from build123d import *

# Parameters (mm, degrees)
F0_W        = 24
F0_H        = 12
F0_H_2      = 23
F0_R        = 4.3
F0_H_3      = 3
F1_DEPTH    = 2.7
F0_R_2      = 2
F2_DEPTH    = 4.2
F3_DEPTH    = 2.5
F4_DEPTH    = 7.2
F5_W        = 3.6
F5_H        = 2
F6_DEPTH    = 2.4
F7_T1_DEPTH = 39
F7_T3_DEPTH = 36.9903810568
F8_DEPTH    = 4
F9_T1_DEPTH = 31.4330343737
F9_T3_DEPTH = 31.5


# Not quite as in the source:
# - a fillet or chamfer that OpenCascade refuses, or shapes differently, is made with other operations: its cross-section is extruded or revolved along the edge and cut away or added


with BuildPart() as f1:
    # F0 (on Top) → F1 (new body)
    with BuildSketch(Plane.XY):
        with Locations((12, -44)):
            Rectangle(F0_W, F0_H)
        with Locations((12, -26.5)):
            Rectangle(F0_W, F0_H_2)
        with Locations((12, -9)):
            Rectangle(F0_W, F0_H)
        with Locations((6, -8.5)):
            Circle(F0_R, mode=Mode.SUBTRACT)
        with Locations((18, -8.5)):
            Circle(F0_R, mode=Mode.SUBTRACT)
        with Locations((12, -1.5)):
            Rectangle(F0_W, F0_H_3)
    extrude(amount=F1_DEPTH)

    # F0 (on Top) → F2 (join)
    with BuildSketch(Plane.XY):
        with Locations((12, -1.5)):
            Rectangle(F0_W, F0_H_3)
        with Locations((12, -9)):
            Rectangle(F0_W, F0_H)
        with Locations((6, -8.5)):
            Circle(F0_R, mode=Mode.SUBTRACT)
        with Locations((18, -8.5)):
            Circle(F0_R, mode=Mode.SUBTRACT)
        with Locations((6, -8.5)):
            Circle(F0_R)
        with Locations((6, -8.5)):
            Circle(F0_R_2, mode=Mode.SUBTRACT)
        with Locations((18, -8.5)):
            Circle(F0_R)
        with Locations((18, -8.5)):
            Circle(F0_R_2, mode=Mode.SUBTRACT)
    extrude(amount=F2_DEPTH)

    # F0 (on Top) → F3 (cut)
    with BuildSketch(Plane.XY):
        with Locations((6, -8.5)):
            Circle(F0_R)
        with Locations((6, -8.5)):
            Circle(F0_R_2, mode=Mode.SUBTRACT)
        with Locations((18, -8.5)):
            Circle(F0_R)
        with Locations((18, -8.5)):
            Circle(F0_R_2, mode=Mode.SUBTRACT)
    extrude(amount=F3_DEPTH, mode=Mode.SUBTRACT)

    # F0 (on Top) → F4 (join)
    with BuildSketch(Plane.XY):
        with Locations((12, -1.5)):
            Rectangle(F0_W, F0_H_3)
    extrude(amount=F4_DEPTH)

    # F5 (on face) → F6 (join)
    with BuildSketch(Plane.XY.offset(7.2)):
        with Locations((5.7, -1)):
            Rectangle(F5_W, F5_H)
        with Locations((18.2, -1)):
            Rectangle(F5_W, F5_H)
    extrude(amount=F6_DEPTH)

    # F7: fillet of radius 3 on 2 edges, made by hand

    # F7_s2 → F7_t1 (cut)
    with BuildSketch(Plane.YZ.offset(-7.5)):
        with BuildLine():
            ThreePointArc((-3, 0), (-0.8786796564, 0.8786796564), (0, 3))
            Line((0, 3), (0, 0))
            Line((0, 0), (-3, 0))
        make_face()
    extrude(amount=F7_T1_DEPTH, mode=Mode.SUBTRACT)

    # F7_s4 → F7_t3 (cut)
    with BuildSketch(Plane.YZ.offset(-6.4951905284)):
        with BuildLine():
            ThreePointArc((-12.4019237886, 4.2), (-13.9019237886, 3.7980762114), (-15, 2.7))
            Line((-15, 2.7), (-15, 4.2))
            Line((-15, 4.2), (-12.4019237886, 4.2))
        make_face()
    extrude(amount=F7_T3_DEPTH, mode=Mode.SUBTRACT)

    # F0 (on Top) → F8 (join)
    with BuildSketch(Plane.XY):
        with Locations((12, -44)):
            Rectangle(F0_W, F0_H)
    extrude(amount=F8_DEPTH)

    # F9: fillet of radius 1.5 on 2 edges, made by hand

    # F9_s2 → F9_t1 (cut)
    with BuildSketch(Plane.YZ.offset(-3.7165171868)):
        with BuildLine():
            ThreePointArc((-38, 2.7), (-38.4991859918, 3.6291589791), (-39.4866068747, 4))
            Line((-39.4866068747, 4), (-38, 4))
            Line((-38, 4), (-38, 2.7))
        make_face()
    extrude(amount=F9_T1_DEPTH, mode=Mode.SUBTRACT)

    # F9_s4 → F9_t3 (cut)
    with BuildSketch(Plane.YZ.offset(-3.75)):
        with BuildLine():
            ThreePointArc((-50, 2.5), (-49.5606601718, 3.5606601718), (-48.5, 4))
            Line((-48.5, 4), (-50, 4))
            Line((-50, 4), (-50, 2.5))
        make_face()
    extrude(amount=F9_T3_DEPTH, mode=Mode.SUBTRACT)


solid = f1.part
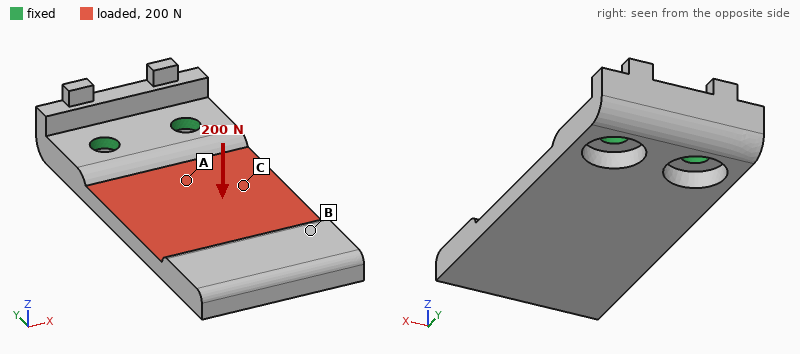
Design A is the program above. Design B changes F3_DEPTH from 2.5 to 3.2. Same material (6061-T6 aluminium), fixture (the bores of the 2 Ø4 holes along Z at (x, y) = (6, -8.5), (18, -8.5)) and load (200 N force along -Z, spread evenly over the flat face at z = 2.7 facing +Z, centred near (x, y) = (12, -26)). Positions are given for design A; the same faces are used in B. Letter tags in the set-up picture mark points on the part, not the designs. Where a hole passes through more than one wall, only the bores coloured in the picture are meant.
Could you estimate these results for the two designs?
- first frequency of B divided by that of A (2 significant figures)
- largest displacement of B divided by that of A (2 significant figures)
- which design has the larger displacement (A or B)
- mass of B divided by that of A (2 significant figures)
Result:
0.87
1.4
B
0.98
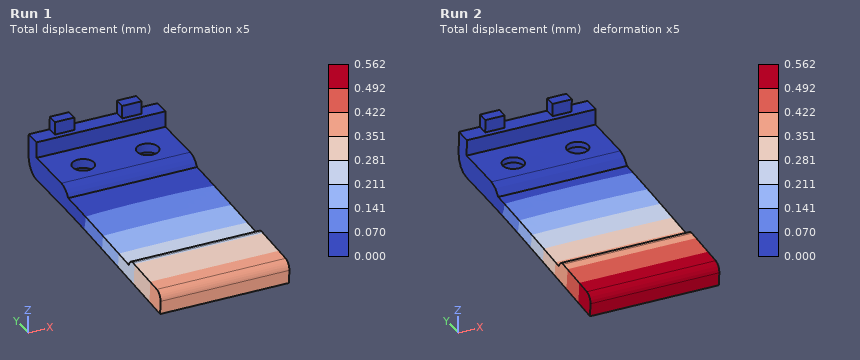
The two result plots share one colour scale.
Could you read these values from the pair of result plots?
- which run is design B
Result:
Run 2
